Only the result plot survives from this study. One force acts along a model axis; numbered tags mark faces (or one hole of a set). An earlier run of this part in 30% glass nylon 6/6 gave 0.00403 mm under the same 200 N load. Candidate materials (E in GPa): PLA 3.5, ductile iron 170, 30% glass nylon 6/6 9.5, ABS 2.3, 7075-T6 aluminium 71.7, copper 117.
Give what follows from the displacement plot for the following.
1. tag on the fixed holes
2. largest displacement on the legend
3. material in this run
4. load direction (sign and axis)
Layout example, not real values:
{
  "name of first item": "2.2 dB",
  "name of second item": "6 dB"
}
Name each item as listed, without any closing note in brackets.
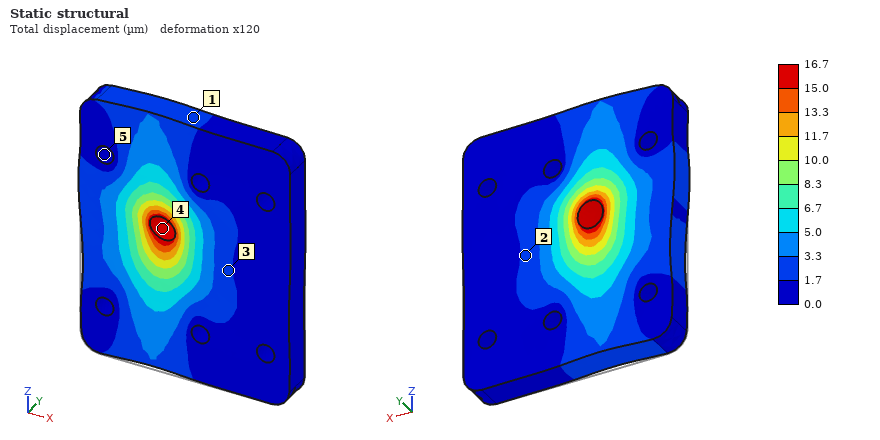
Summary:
{
  "tag on the fixed holes": "5",
  "largest displacement on the legend": "16.7 µm",
  "material in this run": "ABS",
  "load direction": "+Z"
}
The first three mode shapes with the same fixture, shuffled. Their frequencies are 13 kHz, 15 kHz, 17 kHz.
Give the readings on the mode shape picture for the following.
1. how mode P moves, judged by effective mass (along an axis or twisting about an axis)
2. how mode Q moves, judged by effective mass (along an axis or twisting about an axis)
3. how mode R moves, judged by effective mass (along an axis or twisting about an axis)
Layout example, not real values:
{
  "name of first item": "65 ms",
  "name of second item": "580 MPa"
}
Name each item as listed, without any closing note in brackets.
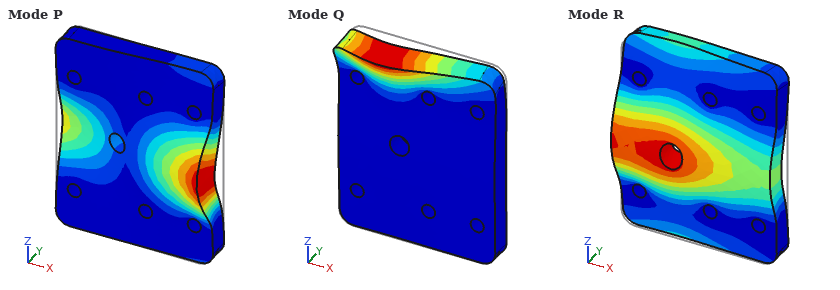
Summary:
{
  "how mode P moves, judged by effective mass": "twisting about Z",
  "how mode Q moves, judged by effective mass": "along Y",
  "how mode R moves, judged by effective mass": "along Y"
}
